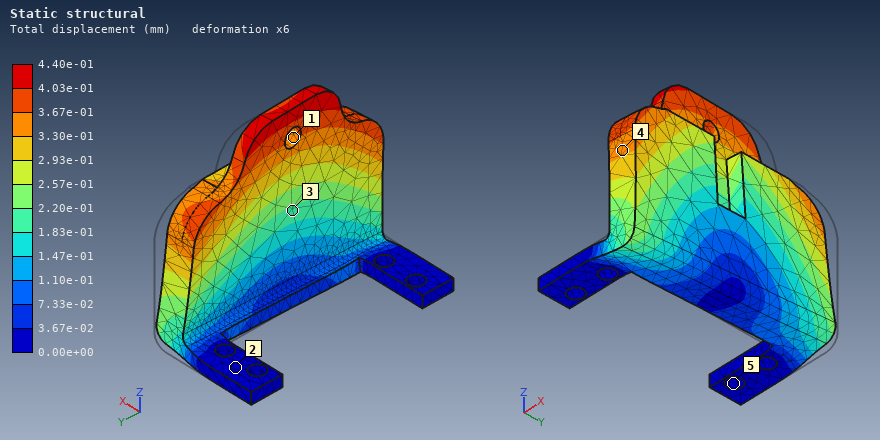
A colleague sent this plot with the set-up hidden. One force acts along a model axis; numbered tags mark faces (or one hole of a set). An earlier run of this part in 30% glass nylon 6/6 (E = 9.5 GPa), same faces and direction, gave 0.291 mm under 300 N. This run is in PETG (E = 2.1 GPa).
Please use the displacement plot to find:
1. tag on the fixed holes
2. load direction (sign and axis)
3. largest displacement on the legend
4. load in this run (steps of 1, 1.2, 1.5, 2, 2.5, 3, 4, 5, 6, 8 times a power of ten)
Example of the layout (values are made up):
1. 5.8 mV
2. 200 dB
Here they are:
1. 5
2. -Y
3. 4.40e-01 mm
4. 100 N
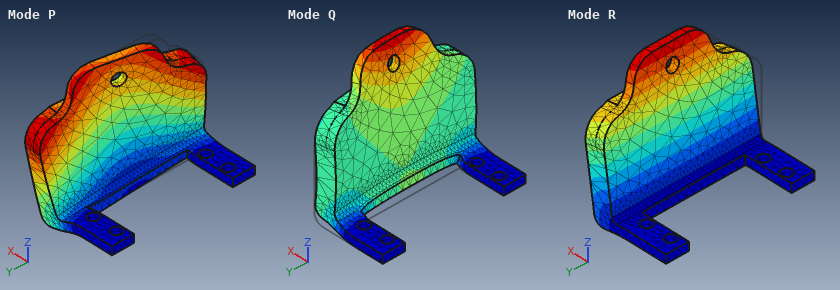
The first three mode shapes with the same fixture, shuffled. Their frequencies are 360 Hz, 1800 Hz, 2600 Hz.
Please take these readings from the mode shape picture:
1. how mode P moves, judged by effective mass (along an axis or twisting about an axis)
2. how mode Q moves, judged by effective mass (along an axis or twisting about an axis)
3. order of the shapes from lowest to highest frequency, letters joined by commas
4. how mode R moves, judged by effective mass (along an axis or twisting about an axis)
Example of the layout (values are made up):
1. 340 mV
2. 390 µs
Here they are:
1. along Y
2. along Z
3. R, P, Q
4. along X
